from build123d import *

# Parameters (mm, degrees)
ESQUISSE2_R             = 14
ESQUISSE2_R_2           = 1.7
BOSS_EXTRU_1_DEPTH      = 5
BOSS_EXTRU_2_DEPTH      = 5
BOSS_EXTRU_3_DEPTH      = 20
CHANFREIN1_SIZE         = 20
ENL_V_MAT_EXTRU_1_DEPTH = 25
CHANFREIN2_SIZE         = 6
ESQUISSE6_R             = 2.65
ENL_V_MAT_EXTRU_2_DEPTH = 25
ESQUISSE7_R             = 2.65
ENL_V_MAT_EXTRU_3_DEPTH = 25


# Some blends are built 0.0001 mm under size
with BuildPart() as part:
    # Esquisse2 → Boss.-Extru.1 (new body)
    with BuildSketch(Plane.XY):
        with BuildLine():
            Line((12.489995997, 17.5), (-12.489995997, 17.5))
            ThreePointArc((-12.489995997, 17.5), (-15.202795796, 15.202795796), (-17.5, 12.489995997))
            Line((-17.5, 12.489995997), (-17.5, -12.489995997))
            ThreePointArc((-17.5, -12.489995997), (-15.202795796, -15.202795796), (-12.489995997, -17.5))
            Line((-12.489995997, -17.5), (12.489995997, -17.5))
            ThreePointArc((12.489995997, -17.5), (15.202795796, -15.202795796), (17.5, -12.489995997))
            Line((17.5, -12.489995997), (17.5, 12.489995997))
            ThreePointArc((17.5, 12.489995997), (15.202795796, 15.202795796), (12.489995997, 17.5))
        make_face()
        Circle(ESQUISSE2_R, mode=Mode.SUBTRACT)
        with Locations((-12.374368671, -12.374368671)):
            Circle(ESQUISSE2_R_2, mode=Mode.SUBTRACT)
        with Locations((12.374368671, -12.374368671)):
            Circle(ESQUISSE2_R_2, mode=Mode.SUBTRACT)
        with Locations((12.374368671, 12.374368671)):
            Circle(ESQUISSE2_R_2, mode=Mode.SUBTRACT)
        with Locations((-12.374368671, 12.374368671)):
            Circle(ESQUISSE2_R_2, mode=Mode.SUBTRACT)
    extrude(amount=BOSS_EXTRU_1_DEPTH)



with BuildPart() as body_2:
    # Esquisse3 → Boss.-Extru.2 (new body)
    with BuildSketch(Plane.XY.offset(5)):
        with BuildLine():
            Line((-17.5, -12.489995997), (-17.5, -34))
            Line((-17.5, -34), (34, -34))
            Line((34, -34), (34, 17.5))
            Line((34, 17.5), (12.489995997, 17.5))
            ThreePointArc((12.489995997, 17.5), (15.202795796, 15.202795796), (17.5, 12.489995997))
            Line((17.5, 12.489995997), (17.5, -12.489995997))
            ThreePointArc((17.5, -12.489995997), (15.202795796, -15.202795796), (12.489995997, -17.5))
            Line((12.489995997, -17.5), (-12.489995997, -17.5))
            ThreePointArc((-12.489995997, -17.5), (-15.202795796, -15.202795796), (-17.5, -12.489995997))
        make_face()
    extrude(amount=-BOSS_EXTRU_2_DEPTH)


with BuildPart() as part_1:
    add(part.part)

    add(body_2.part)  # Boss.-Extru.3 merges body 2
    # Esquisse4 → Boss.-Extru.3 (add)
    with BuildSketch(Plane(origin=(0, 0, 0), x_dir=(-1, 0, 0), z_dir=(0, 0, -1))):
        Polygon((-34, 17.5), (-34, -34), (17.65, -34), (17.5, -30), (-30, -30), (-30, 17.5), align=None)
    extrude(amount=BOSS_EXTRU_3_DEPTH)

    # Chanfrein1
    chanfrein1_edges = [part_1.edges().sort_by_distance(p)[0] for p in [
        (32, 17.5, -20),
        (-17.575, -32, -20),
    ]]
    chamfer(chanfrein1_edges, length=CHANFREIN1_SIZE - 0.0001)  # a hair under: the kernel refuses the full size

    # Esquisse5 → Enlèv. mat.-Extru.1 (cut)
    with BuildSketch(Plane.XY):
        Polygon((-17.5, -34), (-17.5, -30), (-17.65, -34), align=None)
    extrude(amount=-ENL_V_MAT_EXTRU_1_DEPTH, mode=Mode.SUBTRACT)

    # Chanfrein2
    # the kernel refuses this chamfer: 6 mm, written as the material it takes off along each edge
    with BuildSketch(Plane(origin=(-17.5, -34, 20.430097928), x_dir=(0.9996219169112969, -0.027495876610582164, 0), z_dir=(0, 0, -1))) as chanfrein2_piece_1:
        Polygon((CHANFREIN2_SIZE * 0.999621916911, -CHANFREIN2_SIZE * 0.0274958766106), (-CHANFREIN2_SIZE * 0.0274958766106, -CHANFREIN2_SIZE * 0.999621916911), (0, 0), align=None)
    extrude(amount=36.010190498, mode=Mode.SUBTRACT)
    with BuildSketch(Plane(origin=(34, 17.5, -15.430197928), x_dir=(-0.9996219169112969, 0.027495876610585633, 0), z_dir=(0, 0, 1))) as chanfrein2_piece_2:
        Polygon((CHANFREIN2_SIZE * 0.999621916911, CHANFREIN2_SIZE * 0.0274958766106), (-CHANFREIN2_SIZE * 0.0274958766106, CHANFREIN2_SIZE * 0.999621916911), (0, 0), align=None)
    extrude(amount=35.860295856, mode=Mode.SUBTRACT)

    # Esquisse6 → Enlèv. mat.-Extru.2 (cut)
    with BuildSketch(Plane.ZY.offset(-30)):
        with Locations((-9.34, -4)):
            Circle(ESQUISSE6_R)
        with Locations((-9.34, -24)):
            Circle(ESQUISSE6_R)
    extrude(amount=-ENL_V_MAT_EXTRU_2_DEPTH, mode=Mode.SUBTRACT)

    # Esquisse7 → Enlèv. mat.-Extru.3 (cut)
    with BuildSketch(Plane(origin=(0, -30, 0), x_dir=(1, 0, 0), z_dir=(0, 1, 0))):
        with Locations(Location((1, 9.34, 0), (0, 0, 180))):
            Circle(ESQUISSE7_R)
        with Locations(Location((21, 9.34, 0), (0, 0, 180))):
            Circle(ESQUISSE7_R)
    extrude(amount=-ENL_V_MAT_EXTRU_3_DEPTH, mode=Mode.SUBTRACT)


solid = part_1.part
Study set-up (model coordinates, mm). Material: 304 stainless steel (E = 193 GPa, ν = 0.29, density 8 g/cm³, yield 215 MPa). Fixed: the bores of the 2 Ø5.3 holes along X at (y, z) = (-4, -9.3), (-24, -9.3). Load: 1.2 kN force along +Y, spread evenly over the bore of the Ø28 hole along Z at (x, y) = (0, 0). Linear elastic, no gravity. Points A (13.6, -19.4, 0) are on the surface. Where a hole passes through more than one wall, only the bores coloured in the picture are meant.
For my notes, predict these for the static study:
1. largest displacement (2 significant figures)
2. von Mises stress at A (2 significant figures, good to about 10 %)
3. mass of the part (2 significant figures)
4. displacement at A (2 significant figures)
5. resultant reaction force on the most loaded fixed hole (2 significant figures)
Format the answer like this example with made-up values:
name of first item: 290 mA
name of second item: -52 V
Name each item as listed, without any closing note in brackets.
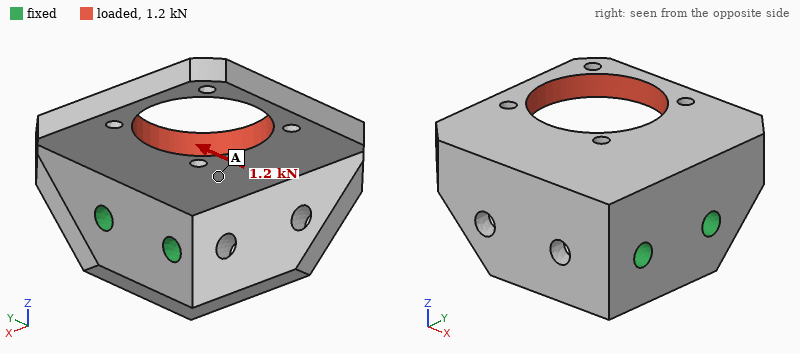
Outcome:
largest displacement: 84 µm
von Mises stress at A: 29 MPa
mass of the part: 130 g
displacement at A: 27 µm
resultant reaction force on the most loaded fixed hole: 1.6 kN
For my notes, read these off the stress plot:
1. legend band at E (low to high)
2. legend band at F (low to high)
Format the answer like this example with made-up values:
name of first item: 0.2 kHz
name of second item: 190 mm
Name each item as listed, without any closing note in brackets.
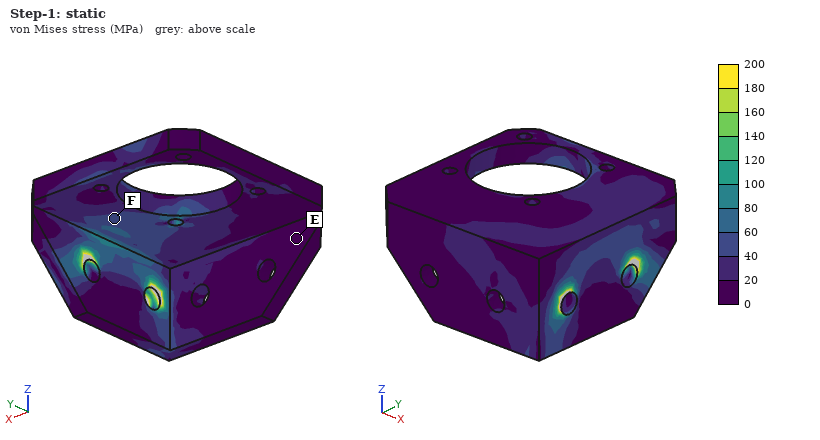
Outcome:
legend band at E: 0 to 20 MPa
legend band at F: 40 to 60 MPa
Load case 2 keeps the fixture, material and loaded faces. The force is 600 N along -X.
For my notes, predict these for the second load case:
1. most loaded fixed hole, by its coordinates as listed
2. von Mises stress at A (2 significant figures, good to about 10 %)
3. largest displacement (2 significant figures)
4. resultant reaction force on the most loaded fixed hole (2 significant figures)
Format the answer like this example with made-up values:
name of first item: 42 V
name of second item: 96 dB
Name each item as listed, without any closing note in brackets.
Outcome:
most loaded fixed hole, by its coordinates as listed: (-4, -9.3)
von Mises stress at A: 9.8 MPa
largest displacement: 35 µm
resultant reaction force on the most loaded fixed hole: 600 N
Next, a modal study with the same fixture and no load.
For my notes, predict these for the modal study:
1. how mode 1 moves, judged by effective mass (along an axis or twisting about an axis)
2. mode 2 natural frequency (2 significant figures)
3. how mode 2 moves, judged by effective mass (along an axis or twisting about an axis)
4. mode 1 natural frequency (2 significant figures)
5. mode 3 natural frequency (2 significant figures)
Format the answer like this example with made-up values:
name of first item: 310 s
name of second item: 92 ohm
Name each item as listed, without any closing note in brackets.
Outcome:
how mode 1 moves, judged by effective mass: along Z
mode 2 natural frequency: 2600 Hz
how mode 2 moves, judged by effective mass: along Y
mode 1 natural frequency: 1700 Hz
mode 3 natural frequency: 4100 Hz
